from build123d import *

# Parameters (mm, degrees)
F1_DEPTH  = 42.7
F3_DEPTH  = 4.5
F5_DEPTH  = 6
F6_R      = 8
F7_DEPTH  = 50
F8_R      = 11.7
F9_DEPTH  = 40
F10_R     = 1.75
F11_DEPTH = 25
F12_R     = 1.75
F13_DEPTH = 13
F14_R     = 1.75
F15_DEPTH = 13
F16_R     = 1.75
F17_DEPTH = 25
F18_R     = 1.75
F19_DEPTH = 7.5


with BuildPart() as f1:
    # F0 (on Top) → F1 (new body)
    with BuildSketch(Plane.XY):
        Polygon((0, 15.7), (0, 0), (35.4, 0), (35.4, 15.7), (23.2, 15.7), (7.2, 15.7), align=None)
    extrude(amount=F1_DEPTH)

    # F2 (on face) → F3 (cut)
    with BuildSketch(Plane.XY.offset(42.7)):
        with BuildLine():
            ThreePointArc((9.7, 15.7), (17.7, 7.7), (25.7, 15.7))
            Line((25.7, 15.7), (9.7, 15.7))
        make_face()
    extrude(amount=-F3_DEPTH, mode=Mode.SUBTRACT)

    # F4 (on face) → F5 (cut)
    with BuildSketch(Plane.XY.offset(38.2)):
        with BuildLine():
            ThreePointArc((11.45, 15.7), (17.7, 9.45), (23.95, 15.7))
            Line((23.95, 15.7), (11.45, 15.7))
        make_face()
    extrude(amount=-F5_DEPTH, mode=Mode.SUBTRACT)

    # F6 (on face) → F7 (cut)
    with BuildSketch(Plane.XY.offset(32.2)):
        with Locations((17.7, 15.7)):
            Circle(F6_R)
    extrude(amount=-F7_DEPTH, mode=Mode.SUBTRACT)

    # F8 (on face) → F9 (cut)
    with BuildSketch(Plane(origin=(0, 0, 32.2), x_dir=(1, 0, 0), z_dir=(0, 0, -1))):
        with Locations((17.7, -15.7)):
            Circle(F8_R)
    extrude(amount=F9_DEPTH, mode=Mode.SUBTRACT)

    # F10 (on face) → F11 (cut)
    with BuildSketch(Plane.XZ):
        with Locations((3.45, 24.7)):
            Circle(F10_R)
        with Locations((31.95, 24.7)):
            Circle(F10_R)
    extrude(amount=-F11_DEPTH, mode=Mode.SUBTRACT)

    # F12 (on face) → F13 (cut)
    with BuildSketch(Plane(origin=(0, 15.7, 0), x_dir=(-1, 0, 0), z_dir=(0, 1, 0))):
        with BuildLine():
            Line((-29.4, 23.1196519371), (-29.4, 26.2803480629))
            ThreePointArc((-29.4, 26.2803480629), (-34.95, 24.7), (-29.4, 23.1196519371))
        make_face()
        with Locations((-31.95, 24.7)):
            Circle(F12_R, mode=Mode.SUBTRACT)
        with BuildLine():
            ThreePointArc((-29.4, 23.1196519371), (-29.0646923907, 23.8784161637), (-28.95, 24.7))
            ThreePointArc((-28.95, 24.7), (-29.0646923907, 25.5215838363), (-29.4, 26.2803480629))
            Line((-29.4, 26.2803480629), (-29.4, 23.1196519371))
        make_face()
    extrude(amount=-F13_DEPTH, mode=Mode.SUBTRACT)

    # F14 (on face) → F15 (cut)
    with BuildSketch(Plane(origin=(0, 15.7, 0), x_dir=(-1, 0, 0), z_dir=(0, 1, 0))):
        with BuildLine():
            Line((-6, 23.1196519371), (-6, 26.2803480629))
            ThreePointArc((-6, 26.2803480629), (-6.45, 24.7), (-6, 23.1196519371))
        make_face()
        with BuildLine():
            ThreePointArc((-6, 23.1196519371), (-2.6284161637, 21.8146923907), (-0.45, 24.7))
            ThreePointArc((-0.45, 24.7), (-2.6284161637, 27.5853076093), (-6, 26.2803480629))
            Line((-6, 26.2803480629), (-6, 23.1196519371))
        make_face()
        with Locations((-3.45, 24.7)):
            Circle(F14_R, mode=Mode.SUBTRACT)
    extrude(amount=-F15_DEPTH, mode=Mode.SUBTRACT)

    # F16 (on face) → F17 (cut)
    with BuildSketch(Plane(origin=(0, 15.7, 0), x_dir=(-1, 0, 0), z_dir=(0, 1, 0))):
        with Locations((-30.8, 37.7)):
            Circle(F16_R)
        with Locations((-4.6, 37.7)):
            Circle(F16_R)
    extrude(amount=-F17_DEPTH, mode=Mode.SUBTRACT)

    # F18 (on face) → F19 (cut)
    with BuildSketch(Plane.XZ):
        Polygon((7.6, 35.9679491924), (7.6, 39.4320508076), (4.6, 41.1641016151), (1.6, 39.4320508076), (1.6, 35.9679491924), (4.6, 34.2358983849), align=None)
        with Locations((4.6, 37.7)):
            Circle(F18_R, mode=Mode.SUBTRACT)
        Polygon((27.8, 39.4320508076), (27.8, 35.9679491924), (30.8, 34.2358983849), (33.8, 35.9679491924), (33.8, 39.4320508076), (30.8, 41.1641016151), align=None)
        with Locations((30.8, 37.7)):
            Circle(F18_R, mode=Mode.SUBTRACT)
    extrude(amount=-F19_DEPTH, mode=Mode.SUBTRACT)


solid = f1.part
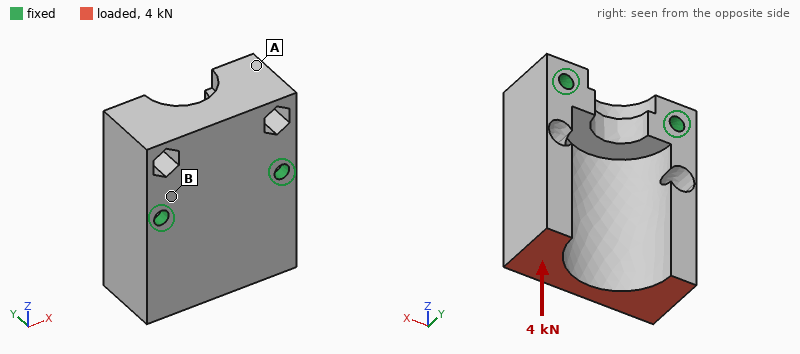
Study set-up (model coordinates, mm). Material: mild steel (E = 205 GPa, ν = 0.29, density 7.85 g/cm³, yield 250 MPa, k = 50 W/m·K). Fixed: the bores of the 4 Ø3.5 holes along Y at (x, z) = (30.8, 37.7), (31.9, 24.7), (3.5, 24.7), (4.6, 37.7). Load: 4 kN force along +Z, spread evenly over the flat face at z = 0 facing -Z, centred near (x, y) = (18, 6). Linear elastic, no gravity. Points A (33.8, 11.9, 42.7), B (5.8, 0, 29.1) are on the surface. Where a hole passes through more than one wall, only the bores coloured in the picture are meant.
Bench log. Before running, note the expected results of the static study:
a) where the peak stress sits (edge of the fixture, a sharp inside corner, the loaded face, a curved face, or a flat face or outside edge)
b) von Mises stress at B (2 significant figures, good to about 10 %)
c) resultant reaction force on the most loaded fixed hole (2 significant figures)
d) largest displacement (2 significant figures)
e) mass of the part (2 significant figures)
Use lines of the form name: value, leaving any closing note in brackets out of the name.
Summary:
where the peak stress sits: a curved face
von Mises stress at B: 18 MPa
resultant reaction force on the most loaded fixed hole: 1.0 kN
largest displacement: 8.5 µm
mass of the part: 110 g
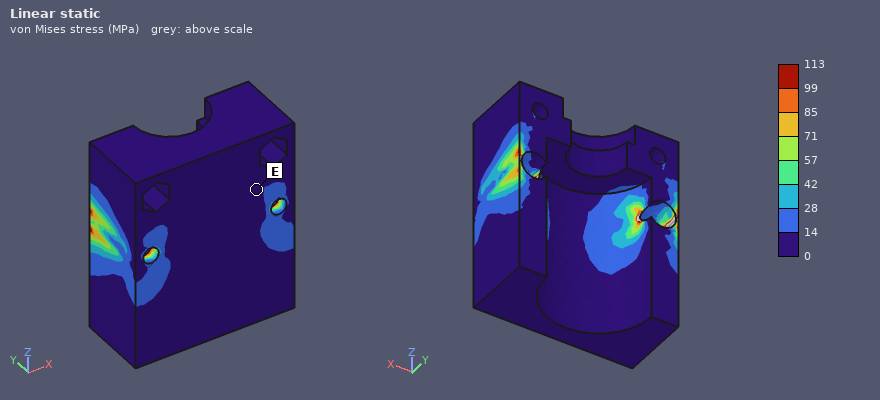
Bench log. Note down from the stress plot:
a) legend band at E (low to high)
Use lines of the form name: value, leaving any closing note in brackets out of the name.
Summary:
legend band at E: 0 to 14 MPa
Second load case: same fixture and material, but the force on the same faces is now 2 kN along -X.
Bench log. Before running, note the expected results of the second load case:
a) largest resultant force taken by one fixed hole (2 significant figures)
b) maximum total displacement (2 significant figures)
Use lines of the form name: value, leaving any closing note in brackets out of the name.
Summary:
largest resultant force taken by one fixed hole: 1.7 kN
maximum total displacement: 12 µm
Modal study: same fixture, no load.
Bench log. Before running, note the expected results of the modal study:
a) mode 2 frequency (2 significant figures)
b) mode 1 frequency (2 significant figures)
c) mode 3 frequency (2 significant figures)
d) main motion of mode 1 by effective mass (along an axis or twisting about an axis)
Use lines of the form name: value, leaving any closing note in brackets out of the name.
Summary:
mode 2 frequency: 11 kHz
mode 1 frequency: 8100 Hz
mode 3 frequency: 15 kHz
main motion of mode 1 by effective mass: along Y
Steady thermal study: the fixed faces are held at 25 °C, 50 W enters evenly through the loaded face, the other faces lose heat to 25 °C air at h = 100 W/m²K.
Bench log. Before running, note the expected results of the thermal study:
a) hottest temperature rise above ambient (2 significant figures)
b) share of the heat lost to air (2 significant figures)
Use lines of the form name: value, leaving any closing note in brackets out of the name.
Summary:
hottest temperature rise above ambient: 80 K
share of the heat lost to air: 32 %
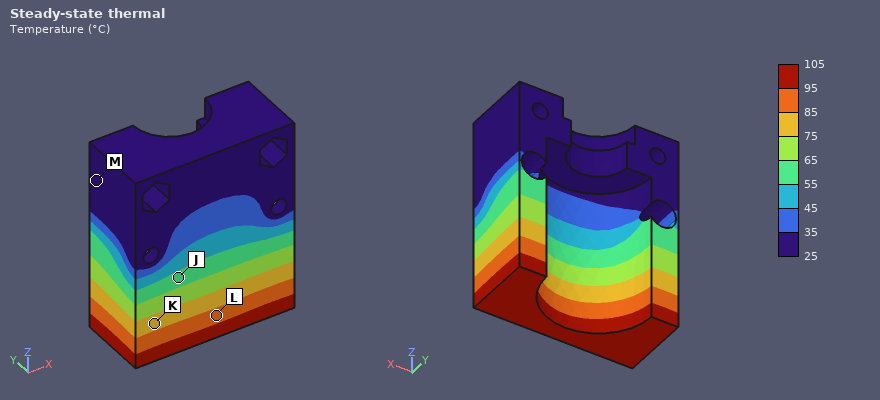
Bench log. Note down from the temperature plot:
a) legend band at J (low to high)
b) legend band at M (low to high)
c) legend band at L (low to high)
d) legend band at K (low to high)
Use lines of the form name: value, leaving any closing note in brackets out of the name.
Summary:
legend band at J: 55 to 65 °C
legend band at M: 25 to 35 °C
legend band at L: 85 to 95 °C
legend band at K: 75 to 85 °C
